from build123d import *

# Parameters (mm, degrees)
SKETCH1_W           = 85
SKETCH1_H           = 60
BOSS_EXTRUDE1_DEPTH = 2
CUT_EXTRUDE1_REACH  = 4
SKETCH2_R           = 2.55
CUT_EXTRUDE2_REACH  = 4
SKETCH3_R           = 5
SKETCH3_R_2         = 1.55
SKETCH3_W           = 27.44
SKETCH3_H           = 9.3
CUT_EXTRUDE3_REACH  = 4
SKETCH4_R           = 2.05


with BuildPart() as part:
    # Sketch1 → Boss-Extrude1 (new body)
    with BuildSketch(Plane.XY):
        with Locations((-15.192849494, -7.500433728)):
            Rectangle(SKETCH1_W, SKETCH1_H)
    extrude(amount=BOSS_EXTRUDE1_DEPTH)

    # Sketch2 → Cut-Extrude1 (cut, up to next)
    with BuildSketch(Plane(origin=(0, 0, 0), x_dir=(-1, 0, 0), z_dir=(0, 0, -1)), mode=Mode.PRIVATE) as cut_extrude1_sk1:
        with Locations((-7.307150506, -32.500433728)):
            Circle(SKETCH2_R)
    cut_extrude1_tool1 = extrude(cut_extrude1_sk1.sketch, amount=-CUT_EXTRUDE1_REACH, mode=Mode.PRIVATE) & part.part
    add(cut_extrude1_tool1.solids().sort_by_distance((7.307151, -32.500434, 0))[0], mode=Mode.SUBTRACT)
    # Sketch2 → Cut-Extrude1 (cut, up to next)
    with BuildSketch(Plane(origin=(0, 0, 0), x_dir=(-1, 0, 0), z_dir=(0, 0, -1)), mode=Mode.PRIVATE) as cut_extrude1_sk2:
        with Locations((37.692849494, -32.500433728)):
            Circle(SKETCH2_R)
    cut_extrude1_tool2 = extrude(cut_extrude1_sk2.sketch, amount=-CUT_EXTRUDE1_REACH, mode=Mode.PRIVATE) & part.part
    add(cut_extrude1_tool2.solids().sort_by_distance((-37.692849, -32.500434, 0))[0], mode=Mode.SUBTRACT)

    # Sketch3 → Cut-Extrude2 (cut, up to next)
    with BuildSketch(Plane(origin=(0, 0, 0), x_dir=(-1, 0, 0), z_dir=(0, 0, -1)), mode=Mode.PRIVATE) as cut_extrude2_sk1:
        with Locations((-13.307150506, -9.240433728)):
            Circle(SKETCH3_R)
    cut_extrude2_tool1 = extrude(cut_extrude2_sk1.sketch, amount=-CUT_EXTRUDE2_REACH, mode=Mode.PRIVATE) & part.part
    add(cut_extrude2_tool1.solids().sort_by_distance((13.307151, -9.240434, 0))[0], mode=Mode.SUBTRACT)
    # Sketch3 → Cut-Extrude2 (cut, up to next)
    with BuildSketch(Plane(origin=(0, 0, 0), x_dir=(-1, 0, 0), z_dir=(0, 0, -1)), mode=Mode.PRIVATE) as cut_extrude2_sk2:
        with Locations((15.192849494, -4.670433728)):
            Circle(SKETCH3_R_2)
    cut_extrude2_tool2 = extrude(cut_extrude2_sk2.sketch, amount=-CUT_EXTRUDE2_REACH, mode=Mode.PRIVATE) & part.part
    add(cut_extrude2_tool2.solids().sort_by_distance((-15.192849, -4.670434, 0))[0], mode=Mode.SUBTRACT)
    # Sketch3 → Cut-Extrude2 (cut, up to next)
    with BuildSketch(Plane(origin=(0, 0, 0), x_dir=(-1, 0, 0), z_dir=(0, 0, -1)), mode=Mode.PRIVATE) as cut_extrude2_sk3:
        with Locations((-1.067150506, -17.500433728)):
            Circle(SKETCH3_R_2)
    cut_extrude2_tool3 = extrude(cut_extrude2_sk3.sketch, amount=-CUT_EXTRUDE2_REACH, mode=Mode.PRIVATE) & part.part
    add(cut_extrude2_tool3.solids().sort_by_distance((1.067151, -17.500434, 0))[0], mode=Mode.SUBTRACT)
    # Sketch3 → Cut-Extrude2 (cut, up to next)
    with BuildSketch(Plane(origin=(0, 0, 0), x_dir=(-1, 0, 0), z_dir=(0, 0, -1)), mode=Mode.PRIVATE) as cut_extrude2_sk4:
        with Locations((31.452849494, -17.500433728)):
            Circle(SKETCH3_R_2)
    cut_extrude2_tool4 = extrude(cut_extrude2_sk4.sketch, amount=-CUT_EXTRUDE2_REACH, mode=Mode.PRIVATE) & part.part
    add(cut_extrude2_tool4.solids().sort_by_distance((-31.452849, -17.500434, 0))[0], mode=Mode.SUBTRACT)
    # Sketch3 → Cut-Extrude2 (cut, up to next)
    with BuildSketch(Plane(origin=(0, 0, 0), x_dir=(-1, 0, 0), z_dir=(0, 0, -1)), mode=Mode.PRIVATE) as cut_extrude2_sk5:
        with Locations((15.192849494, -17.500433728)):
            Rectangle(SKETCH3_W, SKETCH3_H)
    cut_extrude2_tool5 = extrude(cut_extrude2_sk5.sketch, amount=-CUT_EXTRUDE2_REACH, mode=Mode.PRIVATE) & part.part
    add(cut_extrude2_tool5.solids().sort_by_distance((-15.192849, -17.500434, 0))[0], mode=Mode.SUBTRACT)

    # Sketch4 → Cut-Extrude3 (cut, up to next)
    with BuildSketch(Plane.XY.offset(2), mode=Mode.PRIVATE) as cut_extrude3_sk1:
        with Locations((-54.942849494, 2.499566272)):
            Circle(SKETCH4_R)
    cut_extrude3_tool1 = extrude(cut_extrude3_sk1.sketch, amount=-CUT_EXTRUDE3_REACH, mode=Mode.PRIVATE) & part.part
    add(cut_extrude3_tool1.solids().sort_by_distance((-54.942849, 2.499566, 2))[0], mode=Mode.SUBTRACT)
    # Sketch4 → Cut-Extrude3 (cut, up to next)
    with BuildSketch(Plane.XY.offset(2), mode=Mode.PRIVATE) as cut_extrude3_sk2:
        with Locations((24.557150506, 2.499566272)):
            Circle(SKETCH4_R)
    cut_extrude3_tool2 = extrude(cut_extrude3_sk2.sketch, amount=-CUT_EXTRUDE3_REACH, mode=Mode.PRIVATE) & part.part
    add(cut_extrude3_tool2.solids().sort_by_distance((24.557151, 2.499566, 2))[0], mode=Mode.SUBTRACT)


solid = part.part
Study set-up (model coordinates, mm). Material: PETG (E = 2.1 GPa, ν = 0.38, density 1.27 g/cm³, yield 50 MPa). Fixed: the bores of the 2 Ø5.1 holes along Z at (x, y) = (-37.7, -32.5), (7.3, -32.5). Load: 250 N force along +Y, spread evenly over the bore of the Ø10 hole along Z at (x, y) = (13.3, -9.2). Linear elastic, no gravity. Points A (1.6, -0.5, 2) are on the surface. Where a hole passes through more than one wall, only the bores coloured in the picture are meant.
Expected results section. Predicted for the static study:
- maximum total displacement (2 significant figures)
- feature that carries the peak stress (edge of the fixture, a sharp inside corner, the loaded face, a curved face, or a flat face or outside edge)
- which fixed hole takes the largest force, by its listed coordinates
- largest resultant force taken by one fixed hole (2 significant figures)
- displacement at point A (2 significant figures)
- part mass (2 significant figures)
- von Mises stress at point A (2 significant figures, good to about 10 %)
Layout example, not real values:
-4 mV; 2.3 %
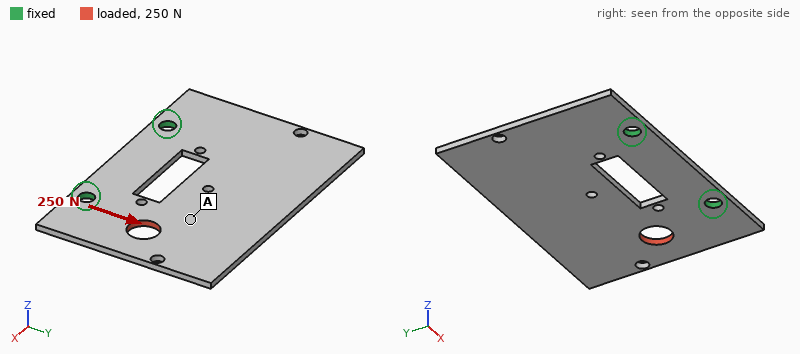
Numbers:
0.21 mm; edge of the fixture; (7.3, -32.5); 270 N; 0.11 mm; 12 g; 2.1 MPa
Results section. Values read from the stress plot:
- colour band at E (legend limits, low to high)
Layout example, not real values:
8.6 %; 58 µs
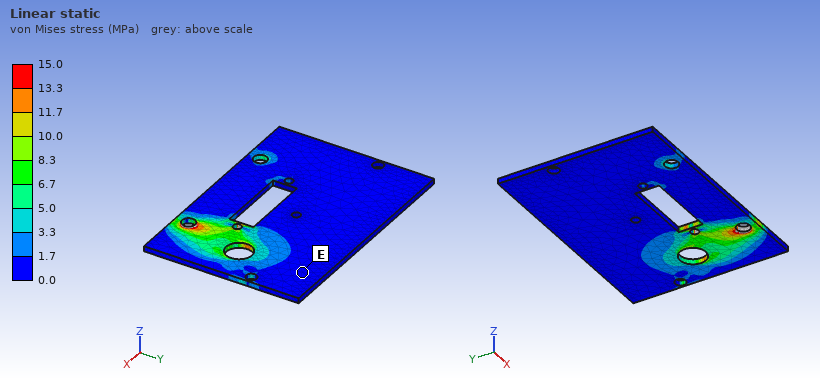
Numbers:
0.0 to 1.7 MPa
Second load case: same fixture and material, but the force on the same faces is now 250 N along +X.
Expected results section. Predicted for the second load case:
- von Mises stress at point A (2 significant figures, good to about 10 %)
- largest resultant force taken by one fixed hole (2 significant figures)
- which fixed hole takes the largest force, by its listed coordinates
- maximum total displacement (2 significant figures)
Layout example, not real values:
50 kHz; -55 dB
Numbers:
4.4 MPa; 180 N; (7.3, -32.5); 0.31 mm
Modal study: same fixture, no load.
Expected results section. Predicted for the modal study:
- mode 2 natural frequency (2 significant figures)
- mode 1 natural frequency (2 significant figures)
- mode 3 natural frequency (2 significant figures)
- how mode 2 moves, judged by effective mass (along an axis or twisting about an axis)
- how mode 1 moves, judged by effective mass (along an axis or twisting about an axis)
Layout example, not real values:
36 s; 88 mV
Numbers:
220 Hz; 110 Hz; 490 Hz; twisting about Y; along Z
